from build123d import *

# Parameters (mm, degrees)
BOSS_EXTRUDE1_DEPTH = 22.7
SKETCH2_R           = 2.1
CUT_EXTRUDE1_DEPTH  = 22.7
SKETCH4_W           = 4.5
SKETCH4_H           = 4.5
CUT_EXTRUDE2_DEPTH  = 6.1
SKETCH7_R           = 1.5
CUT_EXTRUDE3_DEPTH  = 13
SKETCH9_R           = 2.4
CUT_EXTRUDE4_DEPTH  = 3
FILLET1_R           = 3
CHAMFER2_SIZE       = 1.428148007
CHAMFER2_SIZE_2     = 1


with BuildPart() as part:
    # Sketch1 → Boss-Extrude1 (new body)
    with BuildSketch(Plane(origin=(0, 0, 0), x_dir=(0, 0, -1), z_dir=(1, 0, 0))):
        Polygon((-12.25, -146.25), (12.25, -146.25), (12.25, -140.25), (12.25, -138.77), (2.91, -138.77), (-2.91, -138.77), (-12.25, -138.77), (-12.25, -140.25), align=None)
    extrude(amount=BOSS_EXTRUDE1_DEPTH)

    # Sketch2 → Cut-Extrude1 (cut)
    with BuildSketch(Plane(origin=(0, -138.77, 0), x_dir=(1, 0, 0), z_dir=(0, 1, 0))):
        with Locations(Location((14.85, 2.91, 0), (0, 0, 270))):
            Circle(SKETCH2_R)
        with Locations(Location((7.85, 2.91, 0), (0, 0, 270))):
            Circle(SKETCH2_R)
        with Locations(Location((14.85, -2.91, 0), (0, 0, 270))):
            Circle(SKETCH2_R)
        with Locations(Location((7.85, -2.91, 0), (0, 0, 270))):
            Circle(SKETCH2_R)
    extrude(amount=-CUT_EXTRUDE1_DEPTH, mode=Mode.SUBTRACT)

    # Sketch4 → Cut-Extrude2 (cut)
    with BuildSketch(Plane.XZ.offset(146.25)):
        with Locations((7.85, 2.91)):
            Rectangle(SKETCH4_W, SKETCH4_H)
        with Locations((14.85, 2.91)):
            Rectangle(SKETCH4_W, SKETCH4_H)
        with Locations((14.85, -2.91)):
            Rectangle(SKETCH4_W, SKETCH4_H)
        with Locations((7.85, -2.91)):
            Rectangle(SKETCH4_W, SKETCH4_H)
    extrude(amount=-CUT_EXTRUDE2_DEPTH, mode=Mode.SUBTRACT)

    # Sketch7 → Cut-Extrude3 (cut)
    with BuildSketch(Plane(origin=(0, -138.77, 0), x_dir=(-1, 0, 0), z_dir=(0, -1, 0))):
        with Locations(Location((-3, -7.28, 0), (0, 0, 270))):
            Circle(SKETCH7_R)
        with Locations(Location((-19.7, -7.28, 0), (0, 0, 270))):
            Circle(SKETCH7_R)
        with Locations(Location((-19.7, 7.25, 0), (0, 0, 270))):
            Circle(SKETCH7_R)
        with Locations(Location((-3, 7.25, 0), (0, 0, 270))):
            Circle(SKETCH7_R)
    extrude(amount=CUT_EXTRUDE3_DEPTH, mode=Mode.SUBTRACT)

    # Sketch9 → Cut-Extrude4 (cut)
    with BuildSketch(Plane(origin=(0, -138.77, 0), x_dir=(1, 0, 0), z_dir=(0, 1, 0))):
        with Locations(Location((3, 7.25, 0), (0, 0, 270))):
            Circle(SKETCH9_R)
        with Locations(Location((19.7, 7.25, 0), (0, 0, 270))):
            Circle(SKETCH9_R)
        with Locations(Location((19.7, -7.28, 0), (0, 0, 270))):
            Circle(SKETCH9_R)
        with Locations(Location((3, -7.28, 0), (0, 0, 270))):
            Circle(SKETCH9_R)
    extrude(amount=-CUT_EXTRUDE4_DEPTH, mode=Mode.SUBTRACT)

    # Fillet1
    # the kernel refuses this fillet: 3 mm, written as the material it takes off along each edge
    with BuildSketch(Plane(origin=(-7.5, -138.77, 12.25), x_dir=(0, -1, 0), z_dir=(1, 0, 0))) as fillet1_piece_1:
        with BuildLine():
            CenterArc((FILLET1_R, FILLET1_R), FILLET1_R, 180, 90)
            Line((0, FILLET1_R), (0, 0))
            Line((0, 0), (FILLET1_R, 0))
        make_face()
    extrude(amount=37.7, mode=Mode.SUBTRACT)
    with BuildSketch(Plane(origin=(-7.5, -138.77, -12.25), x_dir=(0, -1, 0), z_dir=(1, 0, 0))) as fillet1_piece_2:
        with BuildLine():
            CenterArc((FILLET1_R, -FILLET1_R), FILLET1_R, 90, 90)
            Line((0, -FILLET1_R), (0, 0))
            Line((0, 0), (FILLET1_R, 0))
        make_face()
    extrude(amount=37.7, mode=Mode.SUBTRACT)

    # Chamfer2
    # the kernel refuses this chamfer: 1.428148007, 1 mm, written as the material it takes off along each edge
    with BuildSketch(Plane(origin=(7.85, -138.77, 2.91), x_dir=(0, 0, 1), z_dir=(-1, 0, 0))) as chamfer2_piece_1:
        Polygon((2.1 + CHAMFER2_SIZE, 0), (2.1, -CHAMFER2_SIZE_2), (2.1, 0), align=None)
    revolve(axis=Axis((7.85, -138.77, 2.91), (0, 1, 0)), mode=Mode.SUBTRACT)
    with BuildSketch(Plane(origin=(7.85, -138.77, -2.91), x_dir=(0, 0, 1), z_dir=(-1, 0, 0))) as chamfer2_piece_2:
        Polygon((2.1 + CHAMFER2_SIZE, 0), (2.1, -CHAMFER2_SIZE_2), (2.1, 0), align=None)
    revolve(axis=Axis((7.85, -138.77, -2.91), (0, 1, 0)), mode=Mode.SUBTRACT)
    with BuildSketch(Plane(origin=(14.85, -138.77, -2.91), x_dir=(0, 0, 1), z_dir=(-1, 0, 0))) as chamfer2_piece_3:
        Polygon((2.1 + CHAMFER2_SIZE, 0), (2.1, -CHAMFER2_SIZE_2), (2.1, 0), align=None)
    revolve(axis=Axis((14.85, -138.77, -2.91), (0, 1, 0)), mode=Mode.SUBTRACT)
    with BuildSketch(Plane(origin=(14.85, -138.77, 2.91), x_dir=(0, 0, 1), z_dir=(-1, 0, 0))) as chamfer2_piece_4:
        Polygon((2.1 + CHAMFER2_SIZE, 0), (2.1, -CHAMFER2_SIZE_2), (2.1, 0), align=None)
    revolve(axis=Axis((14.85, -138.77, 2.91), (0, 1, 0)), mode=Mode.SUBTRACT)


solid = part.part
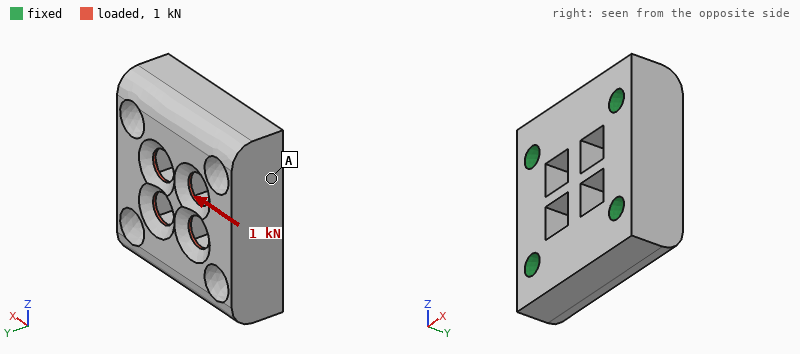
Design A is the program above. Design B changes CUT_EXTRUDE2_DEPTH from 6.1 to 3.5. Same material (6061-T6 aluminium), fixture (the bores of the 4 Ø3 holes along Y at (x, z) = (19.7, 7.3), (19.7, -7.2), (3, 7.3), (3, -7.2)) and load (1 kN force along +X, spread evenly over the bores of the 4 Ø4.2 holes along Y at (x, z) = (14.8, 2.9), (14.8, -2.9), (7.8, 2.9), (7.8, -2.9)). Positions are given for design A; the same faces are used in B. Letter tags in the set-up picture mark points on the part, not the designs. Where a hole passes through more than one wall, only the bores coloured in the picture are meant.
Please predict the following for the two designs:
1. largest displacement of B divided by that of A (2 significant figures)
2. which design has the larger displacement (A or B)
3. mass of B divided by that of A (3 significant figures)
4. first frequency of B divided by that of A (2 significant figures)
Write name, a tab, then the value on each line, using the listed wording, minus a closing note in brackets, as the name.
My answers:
largest displacement of B divided by that of A	0.54
which design has the larger displacement	A
mass of B divided by that of A	1.02
first frequency of B divided by that of A	1.00
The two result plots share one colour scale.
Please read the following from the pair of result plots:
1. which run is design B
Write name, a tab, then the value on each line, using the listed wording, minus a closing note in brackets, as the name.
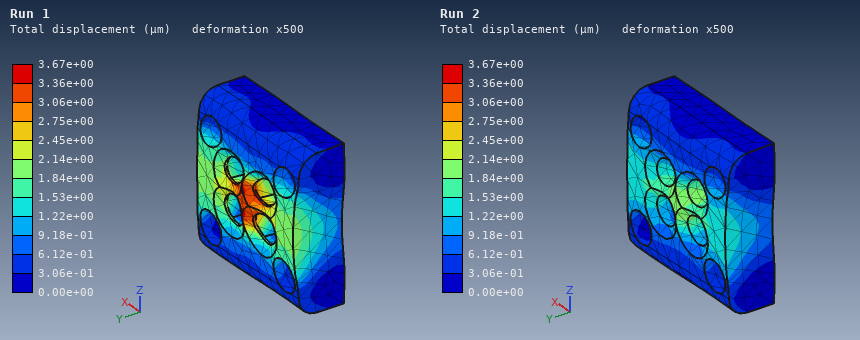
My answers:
which run is design B	Run 2
